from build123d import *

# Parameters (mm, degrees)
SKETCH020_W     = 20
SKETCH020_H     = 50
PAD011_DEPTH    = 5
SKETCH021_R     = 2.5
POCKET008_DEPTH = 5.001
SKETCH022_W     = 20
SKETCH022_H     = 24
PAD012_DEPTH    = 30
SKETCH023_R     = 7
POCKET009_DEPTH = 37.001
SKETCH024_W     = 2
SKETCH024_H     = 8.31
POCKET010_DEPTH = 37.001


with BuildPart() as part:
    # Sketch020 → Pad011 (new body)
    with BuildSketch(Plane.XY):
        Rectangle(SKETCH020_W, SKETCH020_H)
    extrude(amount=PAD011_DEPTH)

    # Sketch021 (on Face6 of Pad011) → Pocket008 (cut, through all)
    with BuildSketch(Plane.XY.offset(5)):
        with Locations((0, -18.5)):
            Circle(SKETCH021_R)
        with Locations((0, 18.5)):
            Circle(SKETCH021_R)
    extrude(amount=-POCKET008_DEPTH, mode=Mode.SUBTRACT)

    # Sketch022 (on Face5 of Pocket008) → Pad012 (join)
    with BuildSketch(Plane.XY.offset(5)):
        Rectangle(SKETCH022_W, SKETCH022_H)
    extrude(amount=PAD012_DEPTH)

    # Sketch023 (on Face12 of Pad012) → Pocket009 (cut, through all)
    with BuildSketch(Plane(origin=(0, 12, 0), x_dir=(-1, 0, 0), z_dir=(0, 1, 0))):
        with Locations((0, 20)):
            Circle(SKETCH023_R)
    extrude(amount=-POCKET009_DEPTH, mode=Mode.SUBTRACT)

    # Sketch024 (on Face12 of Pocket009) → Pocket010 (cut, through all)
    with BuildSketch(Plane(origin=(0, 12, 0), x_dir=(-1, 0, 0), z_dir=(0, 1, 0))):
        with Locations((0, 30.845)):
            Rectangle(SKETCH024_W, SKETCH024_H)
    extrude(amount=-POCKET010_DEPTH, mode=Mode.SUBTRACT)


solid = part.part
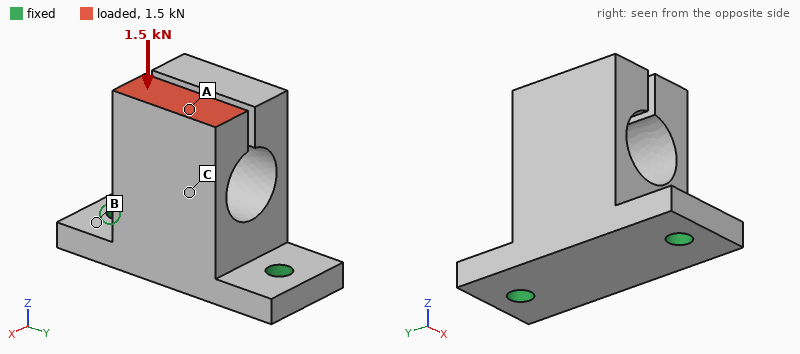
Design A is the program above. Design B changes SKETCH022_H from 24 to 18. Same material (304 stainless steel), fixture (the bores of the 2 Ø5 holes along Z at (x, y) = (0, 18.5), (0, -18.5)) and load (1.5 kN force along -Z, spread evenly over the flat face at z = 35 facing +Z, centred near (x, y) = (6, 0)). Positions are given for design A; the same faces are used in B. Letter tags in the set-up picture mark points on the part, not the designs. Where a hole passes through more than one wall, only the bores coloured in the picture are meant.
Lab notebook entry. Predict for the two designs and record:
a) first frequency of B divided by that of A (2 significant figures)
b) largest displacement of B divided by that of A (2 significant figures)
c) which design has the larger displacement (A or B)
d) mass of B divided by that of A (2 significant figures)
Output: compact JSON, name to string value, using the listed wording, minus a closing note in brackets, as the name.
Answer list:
{"first frequency of B divided by that of A": "0.99", "largest displacement of B divided by that of A": "1.4", "which design has the larger displacement": "B", "mass of B divided by that of A": "0.83"}
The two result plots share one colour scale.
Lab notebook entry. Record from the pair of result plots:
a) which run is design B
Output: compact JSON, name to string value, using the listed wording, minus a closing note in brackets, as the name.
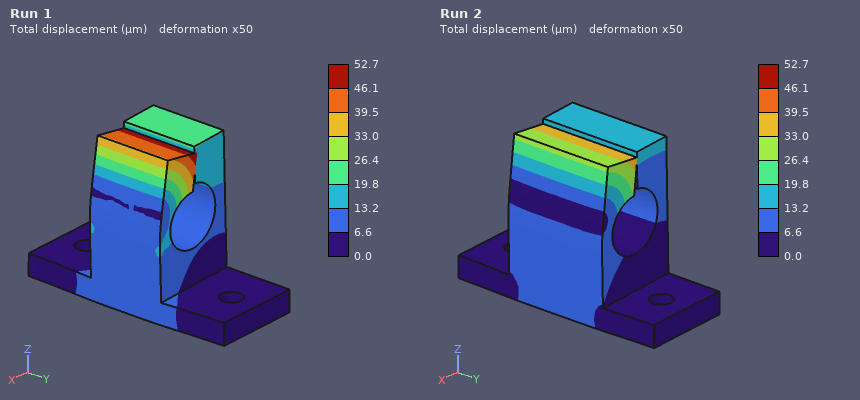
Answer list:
{"which run is design B": "Run 1"}
